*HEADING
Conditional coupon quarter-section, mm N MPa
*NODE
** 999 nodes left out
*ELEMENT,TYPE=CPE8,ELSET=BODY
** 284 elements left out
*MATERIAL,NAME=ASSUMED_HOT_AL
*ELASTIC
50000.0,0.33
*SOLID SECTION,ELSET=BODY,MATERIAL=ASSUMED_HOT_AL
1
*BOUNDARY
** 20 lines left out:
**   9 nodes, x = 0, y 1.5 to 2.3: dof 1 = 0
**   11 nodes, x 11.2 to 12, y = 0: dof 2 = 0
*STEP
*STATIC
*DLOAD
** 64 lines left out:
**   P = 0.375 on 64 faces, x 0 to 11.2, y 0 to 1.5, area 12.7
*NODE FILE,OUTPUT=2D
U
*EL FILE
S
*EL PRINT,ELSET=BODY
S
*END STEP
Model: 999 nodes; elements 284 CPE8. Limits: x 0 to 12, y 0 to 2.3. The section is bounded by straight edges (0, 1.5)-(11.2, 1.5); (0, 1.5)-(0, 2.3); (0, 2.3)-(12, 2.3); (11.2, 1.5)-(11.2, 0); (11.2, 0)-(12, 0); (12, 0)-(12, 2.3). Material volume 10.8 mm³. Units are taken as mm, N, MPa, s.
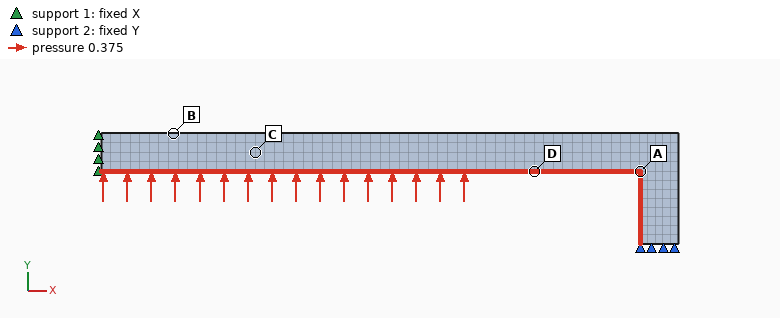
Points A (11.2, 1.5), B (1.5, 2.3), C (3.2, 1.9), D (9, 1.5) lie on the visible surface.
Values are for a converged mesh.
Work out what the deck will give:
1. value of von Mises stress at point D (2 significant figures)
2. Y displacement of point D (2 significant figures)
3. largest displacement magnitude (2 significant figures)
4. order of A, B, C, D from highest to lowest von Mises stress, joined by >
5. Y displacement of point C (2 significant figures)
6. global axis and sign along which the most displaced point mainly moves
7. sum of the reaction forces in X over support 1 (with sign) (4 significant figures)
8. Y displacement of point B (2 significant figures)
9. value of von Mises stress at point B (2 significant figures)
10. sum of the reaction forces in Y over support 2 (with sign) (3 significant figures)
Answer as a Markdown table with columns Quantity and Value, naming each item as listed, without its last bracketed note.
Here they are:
| Quantity | Value |
|---|---|
| value of von Mises stress at point D | 40 MPa |
| Y displacement of point D | 0.042 mm |
| largest displacement magnitude | 0.18 mm |
| order of A, B, C, D from highest to lowest von Mises stress, joined by > | A > B > D > C |
| Y displacement of point C | 0.16 mm |
| global axis and sign along which the most displaced point mainly moves | +Y |
| sum of the reaction forces in X over support 1 (with sign) | -0.5625 N |
| Y displacement of point B | 0.17 mm |
| value of von Mises stress at point B | 84 MPa |
| sum of the reaction forces in Y over support 2 (with sign) | -4.20 N |
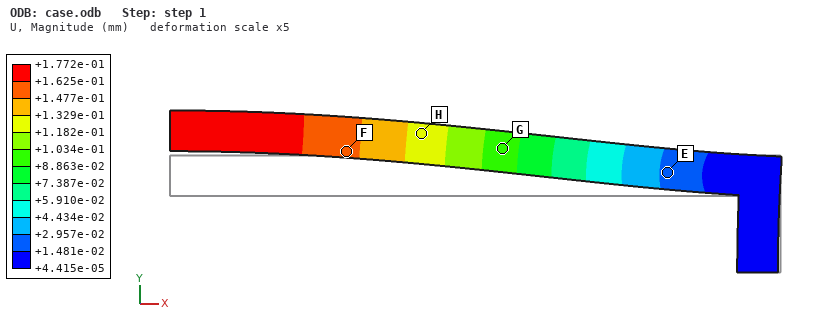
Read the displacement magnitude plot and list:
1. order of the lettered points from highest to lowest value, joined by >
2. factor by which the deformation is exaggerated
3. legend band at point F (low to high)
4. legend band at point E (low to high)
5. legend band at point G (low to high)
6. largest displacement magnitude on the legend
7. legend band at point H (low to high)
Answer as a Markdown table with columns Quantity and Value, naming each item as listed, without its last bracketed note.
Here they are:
| Quantity | Value |
|---|---|
| order of the lettered points from highest to lowest value, joined by > | F > H > G > E |
| factor by which the deformation is exaggerated | 5 |
| legend band at point F | +1.477e-01 to +1.625e-01 mm |
| legend band at point E | +1.481e-02 to +2.957e-02 mm |
| legend band at point G | +8.863e-02 to +1.034e-01 mm |
| largest displacement magnitude on the legend | +1.772e-01 mm |
| legend band at point H | +1.182e-01 to +1.329e-01 mm |
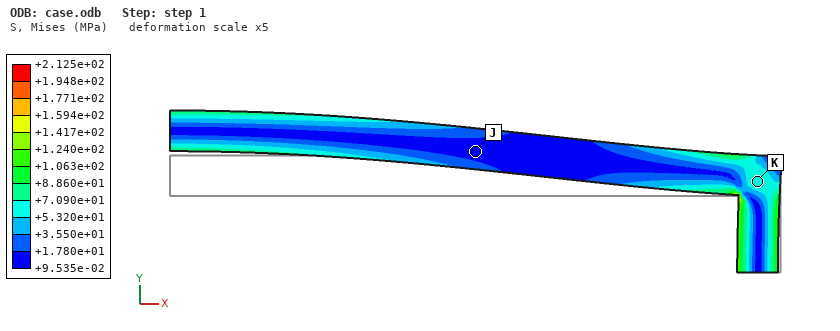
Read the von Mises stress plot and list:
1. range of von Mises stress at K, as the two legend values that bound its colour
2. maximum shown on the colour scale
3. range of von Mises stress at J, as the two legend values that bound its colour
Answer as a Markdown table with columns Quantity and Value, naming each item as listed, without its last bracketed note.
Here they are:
| Quantity | Value |
|---|---|
| range of von Mises stress at K, as the two legend values that bound its colour | +5.320e+01 to +7.090e+01 MPa |
| maximum shown on the colour scale | +2.125e+02 MPa |
| range of von Mises stress at J, as the two legend values that bound its colour | +9.535e-02 to +1.780e+01 MPa |
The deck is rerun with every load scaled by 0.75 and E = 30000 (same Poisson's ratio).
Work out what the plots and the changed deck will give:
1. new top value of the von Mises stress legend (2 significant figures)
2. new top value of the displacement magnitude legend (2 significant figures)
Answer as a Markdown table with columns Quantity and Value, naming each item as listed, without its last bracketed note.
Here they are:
| Quantity | Value |
|---|---|
| new top value of the von Mises stress legend | 160 MPa |
| new top value of the displacement magnitude legend | 0.22 mm |
